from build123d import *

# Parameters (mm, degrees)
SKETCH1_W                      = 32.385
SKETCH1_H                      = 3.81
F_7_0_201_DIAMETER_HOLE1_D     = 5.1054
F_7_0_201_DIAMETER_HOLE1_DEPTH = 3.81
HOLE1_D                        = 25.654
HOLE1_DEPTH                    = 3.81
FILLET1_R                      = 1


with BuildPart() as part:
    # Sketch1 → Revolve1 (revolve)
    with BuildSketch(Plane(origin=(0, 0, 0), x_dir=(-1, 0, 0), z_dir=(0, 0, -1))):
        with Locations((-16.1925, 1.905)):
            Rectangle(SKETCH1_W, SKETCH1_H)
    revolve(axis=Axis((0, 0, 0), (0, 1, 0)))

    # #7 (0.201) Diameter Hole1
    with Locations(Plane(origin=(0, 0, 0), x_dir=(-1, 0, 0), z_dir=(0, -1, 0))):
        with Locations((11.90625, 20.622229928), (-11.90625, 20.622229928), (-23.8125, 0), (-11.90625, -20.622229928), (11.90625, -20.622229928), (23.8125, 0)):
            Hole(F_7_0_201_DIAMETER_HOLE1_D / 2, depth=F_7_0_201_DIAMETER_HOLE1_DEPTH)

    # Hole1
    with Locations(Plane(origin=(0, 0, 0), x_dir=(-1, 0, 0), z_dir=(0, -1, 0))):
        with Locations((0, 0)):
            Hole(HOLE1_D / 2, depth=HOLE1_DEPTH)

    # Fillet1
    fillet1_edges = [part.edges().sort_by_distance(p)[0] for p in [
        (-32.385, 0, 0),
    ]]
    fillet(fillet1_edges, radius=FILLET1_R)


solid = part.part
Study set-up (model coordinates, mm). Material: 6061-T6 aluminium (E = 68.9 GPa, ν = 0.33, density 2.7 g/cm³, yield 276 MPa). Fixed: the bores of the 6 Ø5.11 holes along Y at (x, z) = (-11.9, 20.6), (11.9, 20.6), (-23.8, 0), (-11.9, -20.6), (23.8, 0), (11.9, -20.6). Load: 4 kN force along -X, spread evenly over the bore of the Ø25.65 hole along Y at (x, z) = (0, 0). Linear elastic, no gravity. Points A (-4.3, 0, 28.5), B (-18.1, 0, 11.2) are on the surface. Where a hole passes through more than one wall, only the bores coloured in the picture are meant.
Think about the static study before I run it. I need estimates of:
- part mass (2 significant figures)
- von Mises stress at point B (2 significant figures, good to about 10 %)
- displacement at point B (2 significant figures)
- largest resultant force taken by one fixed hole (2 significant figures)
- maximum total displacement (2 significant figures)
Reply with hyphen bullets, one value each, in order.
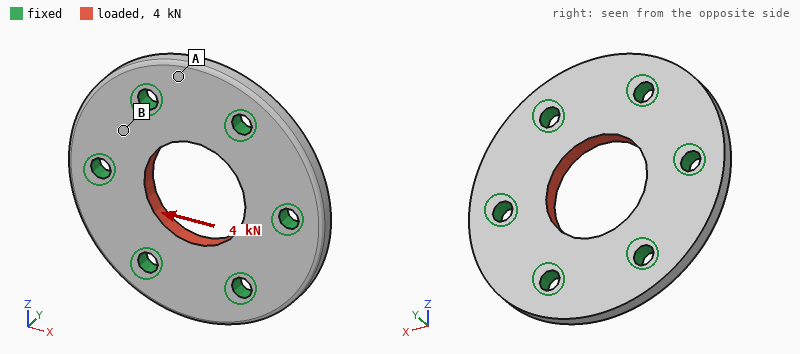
- 27 g
- 5.6 MPa
- 1.7 µm
- 920 N
- 3.1 µm
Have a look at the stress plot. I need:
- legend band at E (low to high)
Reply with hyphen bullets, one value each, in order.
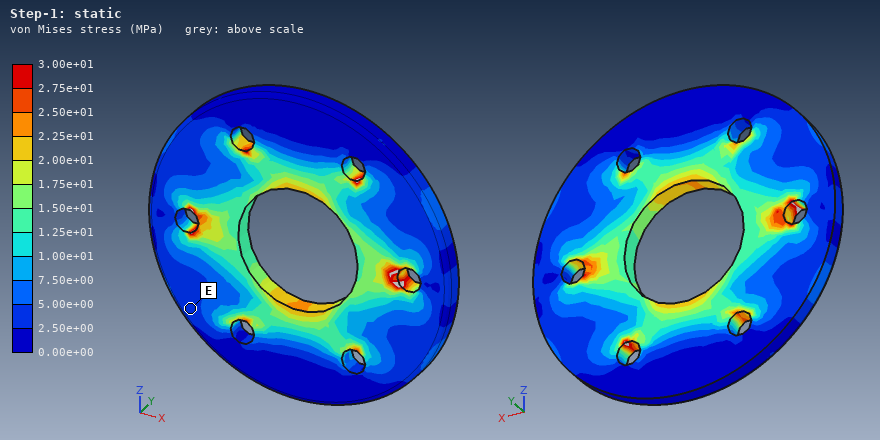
- 2.50e+00 to 5.00e+00 MPa
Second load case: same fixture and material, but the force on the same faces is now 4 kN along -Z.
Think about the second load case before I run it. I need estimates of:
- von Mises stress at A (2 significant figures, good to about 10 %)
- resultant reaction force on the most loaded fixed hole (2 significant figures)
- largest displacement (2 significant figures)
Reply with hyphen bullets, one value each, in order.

- 4.8 MPa
- 820 N
- 3.2 µm
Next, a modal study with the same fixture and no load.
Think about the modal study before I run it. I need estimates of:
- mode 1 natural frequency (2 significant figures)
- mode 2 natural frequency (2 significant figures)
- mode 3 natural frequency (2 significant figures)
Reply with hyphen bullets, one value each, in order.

- 23 kHz
- 23 kHz
- 23 kHz
